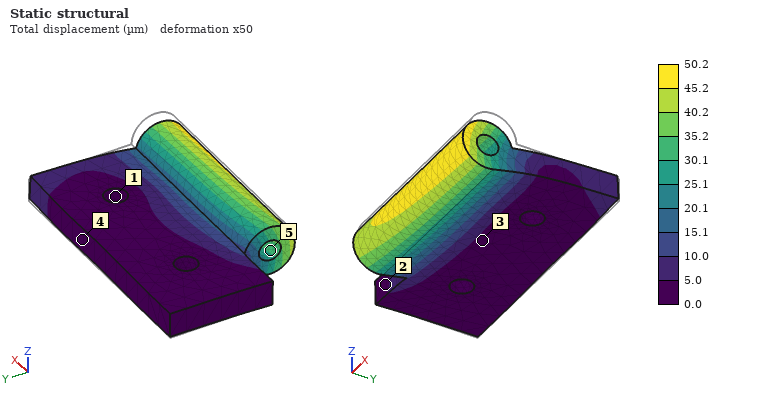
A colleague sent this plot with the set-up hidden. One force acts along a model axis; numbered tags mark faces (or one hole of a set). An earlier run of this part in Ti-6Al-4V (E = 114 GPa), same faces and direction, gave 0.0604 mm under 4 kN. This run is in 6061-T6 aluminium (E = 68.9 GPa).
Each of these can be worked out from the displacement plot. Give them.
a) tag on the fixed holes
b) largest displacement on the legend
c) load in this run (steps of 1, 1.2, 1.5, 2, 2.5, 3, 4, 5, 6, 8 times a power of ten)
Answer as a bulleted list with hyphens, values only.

- 1
- 50.2 µm
- 2 kN
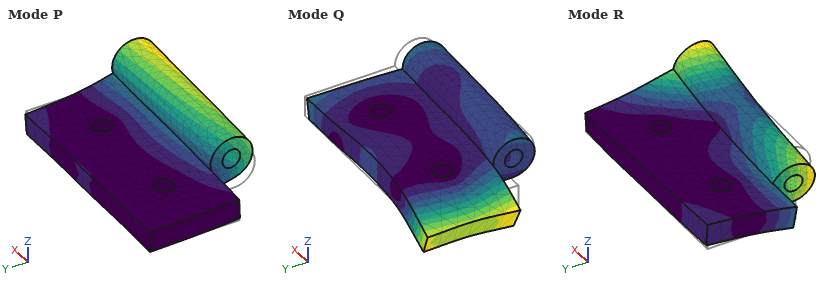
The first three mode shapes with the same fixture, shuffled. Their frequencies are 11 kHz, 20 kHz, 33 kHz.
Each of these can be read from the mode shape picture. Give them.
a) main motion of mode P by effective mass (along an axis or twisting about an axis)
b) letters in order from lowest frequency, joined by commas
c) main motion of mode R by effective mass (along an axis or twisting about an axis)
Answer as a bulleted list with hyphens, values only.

- along Z
- P, R, Q
- twisting about Y
